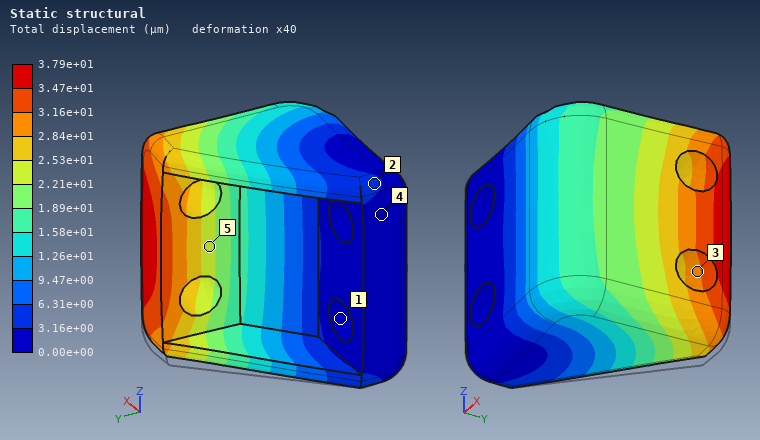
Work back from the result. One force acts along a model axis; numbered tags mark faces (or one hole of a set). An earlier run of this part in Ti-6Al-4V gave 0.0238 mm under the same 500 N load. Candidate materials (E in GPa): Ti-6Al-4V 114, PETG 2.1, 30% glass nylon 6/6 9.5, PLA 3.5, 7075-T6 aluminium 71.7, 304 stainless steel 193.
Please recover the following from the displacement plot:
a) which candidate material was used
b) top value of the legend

7075-T6 aluminium
3.79e+01 µm
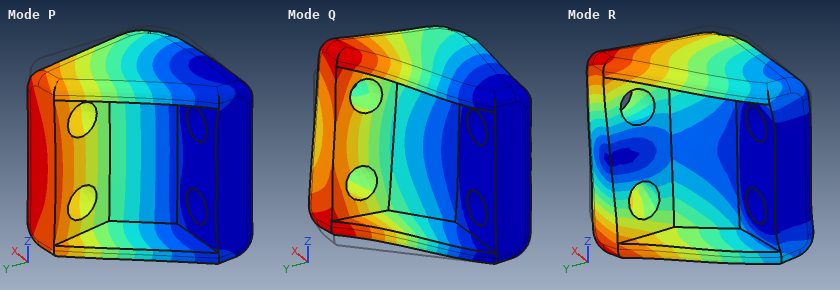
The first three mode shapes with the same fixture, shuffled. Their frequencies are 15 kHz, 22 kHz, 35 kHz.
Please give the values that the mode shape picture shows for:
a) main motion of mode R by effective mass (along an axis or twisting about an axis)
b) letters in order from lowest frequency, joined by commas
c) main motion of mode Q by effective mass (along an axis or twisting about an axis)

along Z
P, Q, R
along Z
